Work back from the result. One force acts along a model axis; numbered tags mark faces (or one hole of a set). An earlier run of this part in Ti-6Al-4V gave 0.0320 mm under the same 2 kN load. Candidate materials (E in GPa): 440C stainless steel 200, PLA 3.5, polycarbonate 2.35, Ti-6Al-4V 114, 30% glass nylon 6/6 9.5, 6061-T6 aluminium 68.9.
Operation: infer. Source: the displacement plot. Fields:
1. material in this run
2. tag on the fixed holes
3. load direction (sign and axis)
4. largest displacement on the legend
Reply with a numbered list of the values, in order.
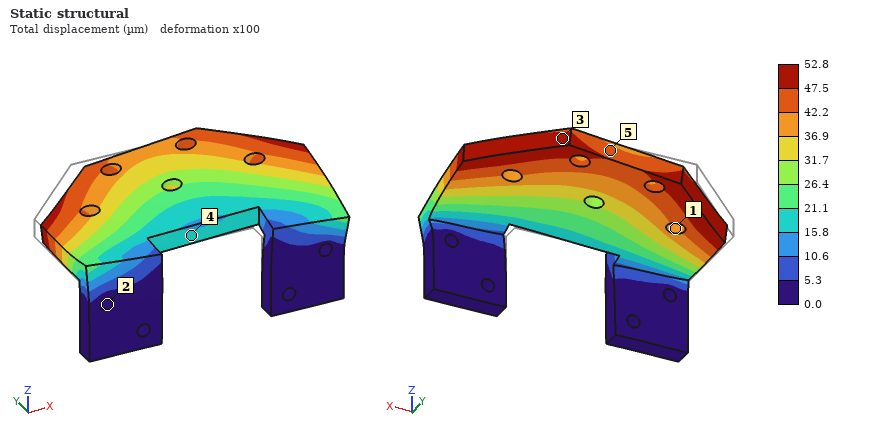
1. 6061-T6 aluminium
2. 2
3. +X
4. 52.8 µm
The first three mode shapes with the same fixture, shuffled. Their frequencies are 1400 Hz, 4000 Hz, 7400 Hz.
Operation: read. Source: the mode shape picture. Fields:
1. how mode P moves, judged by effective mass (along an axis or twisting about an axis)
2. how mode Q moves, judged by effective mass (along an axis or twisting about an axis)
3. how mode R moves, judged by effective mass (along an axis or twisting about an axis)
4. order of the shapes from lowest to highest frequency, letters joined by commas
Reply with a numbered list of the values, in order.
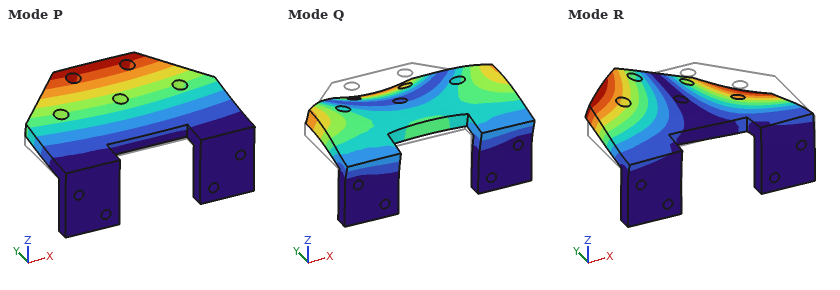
1. along Z
2. along Y
3. twisting about Y
4. P, R, Q
